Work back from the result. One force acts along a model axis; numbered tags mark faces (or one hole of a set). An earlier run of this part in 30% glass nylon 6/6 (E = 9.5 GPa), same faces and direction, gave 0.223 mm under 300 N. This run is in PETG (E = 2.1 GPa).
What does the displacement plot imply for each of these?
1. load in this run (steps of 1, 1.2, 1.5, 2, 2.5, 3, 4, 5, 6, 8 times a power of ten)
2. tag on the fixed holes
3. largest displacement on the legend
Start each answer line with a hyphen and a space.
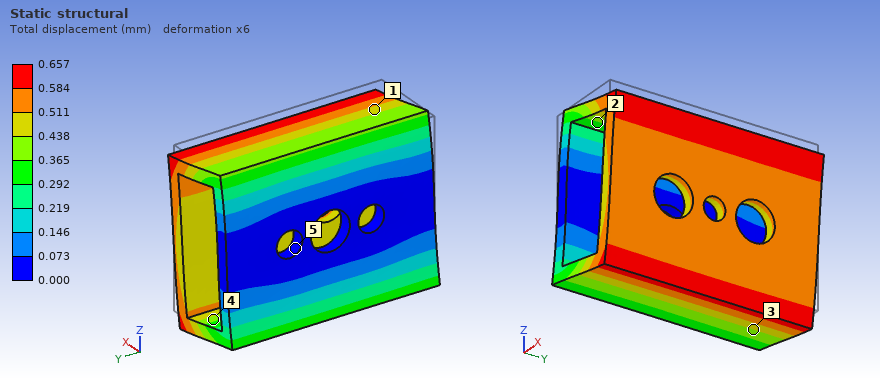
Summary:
- 200 N
- 5
- 0.657 mm
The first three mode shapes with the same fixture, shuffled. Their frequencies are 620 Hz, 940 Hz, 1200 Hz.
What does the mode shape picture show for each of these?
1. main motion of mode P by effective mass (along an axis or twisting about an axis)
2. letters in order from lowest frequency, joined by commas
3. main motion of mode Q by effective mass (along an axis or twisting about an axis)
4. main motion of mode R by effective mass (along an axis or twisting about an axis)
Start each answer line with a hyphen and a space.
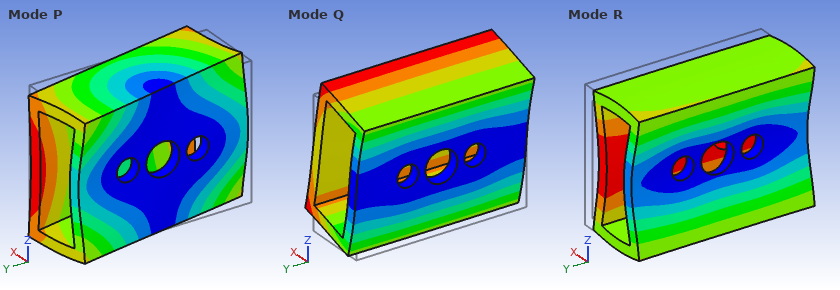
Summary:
- along Y
- Q, P, R
- along Z
- along X
